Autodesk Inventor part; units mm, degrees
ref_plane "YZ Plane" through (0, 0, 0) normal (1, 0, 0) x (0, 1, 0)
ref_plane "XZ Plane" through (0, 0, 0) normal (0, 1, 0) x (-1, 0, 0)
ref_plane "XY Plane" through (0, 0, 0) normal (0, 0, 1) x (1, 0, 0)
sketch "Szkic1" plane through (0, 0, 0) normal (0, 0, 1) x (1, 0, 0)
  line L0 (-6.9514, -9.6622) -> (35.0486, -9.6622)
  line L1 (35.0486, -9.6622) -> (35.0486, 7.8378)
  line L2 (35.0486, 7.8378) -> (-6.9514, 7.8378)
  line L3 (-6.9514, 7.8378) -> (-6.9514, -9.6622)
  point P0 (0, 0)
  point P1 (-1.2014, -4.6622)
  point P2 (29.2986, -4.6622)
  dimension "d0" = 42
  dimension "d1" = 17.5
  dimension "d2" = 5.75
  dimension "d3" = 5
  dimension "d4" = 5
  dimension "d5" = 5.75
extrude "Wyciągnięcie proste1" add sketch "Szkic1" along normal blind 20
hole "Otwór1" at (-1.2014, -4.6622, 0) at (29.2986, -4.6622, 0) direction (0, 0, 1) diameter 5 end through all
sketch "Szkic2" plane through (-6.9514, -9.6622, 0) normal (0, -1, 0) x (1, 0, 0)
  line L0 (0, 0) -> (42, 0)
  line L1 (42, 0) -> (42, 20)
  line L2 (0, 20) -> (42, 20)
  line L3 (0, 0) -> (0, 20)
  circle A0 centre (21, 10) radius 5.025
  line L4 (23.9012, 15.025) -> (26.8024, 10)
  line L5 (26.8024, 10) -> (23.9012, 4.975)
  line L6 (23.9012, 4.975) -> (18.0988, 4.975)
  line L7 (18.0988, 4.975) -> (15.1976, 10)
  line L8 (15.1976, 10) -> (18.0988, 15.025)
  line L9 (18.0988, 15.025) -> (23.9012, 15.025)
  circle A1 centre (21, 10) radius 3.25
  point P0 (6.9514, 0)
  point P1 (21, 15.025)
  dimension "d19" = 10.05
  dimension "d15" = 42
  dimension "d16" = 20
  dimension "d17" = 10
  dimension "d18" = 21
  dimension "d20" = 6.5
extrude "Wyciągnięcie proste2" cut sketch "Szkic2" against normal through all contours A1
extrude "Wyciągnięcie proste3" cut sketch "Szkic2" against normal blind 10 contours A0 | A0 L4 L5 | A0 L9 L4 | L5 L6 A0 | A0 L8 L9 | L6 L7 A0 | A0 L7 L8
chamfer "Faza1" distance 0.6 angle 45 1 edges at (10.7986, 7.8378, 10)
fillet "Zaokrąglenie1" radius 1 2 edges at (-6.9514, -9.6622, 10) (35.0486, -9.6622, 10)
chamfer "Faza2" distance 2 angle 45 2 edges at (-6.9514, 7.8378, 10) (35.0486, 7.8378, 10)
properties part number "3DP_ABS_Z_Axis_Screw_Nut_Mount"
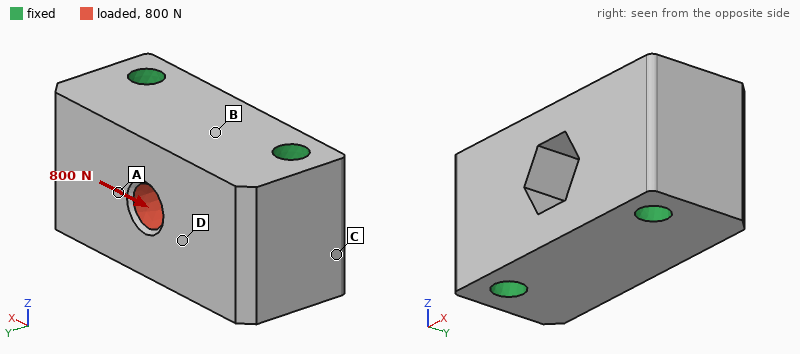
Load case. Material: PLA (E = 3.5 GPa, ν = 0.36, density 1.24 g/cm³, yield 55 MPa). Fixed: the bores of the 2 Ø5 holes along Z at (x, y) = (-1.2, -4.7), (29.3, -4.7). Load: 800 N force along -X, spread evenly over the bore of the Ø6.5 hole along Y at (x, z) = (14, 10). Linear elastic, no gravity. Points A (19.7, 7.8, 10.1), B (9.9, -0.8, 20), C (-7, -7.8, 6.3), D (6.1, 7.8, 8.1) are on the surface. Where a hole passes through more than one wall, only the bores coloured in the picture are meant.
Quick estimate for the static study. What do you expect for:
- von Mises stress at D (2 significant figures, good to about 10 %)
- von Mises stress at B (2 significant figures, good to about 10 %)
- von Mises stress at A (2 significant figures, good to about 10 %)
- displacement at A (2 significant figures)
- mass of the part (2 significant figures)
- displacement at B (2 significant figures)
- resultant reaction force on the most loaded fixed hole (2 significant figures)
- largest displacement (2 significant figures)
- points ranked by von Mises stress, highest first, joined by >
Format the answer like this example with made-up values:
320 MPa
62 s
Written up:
3.0 MPa
1.6 MPa
3.8 MPa
15 µm
16 g
5.1 µm
440 N
18 µm
A > D > B > C
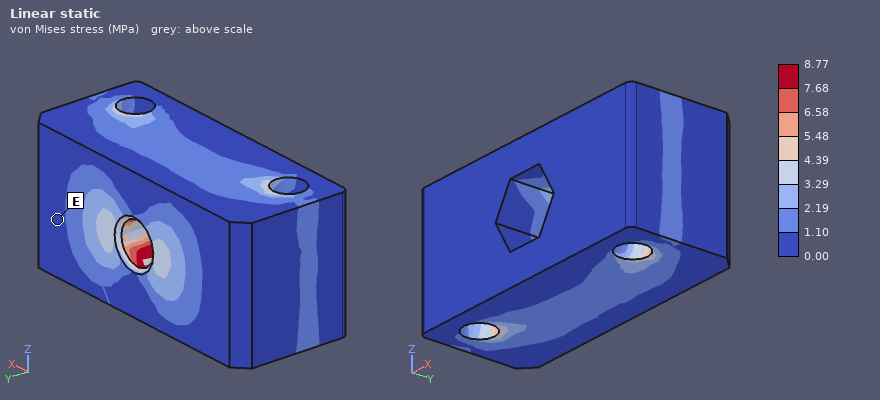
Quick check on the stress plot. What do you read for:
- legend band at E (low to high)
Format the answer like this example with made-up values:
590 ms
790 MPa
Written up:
0.00 to 1.10 MPa
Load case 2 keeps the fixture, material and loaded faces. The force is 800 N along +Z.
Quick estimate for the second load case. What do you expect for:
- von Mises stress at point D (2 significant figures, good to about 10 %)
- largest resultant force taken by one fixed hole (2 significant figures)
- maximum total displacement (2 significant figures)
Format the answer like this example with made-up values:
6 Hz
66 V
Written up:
3.7 MPa
400 N
39 µm
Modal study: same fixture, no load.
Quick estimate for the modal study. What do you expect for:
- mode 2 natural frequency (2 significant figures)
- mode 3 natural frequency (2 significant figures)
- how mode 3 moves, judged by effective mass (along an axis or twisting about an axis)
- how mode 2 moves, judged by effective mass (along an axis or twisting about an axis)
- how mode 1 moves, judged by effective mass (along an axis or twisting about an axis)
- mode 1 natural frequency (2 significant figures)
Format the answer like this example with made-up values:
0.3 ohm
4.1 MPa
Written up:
13 kHz
17 kHz
along X
along Y
along Z
13 kHz
